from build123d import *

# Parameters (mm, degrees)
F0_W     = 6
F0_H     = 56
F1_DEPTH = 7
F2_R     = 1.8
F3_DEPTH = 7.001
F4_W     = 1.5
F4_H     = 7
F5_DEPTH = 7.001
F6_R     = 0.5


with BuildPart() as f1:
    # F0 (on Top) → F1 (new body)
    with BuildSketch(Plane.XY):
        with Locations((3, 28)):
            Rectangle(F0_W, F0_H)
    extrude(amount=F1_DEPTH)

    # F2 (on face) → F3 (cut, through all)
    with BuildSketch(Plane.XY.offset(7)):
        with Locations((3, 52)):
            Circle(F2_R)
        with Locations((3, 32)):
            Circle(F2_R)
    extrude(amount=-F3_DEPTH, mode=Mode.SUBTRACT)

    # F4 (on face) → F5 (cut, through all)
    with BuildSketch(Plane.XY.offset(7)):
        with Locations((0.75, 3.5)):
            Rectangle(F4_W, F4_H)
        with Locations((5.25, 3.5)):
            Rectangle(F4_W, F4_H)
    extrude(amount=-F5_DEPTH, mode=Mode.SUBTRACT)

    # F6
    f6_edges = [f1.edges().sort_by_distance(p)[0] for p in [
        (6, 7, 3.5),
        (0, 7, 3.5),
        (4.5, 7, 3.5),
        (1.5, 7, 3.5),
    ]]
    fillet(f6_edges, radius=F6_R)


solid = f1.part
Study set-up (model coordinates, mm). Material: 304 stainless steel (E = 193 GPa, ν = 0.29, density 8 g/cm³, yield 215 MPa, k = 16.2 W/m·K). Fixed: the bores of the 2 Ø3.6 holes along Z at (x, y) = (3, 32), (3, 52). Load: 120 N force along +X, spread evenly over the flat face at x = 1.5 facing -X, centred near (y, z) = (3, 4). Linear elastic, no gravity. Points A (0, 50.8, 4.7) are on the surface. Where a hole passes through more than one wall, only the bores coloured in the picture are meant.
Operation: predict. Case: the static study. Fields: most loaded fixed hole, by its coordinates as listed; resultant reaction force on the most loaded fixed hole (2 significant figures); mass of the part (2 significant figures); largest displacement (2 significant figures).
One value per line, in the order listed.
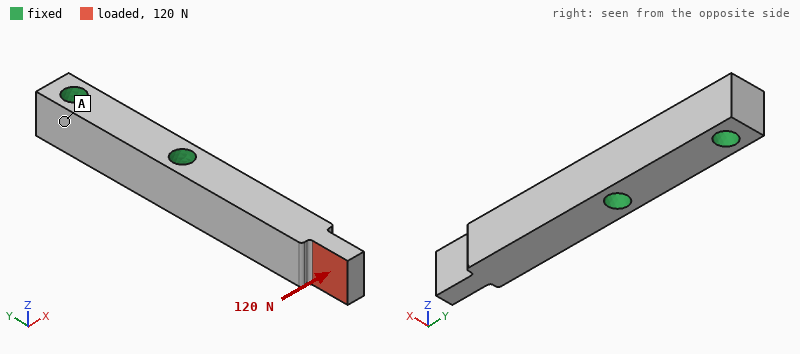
(3, 32)
130 N
16 g
48 µm
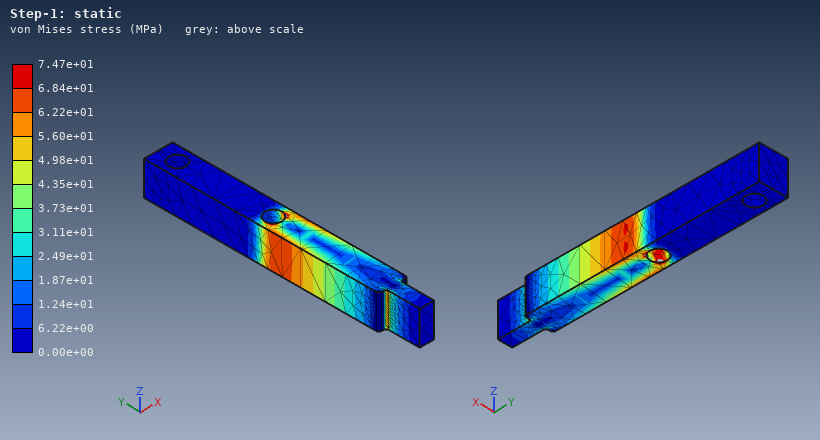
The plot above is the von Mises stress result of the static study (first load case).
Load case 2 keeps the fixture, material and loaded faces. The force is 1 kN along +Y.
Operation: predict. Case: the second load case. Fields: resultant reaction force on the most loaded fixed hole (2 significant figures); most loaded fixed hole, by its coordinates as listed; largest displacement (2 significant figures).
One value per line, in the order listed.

990 N
(3, 32)
41 µm
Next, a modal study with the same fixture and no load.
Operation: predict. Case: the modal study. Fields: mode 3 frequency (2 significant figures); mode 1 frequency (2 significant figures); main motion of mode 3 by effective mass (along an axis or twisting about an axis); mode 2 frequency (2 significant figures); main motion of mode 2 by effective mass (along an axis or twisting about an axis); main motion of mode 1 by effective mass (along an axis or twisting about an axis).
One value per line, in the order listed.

27 kHz
5600 Hz
twisting about Y
6800 Hz
along Z
along X
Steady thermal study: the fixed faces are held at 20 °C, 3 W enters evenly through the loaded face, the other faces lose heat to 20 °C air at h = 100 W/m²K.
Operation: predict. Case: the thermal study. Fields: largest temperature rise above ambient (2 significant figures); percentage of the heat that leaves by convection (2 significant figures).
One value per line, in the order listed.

77 K
68 %
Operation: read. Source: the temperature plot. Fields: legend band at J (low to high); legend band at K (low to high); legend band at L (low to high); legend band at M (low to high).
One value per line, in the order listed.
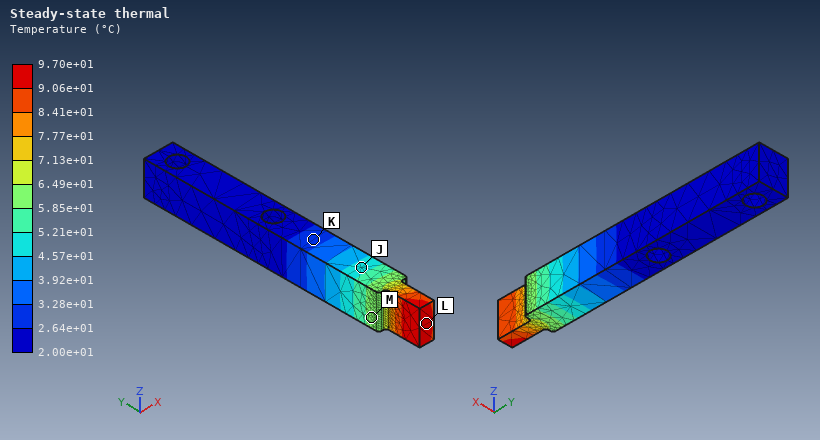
4.57e+01 to 5.21e+01 °C
2.64e+01 to 3.28e+01 °C
9.06e+01 to 9.70e+01 °C
5.85e+01 to 6.49e+01 °C
